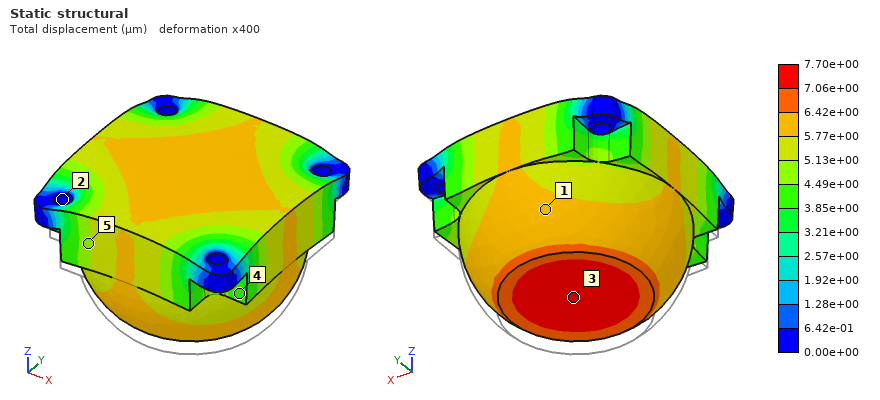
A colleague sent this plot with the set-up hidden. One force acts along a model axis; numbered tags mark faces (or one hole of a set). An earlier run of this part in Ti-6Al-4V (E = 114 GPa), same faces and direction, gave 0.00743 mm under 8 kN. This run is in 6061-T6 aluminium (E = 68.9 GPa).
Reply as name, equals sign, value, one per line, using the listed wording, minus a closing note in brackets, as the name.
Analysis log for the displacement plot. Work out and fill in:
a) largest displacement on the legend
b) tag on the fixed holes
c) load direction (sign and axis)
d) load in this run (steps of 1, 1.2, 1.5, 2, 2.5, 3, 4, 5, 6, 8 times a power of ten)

largest displacement on the legend = 7.70e+00 µm
tag on the fixed holes = 2
load direction = +Z
load in this run = 5 kN
